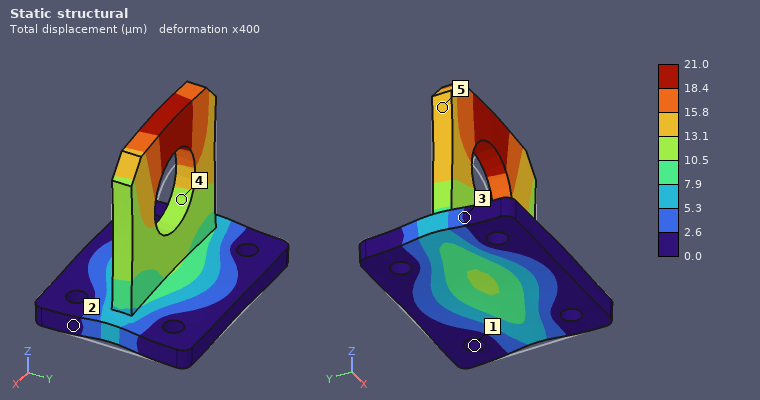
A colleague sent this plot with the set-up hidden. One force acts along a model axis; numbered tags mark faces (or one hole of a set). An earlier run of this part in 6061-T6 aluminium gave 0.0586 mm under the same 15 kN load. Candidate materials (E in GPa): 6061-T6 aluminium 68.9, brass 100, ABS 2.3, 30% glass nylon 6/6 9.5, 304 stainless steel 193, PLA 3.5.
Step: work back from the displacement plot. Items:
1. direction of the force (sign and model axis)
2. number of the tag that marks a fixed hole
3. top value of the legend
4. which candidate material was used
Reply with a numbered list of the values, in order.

1. +Z
2. 1
3. 21.0 µm
4. 304 stainless steel
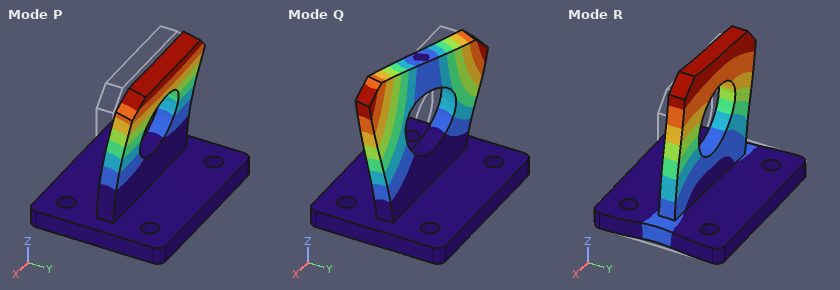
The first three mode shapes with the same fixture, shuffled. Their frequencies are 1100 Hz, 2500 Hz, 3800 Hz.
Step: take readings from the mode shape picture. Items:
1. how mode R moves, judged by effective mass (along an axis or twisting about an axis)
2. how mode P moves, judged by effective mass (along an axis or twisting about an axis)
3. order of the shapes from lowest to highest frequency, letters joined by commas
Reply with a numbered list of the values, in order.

1. along X
2. along Y
3. P, Q, R
